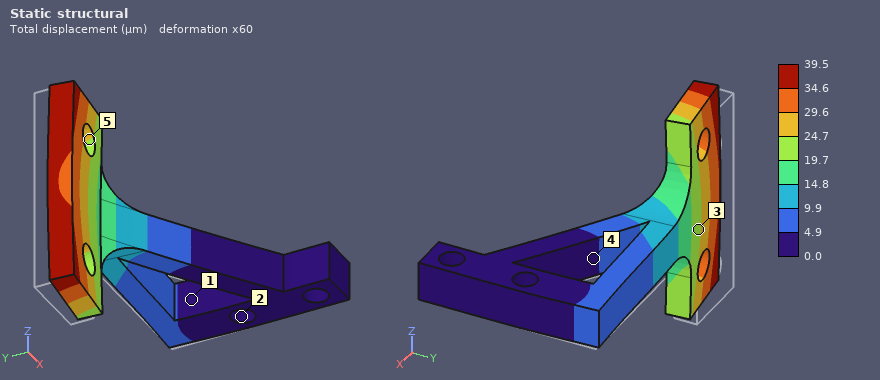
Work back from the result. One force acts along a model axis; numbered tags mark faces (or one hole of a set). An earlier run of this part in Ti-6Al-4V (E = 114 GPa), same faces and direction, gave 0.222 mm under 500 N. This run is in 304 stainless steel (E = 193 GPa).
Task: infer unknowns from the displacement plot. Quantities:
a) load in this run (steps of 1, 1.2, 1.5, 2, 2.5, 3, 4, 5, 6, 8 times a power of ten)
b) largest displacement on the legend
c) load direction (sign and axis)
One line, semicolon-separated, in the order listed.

150 N; 39.5 µm; -Y
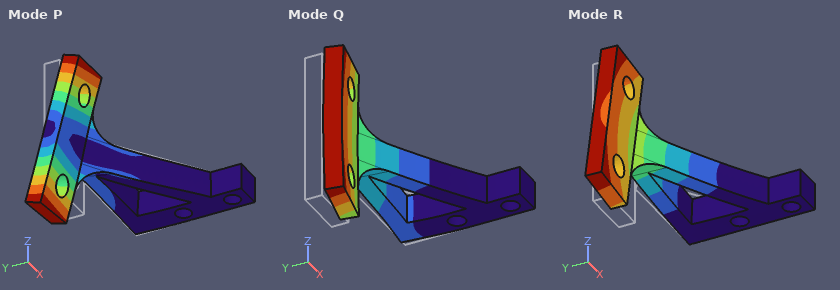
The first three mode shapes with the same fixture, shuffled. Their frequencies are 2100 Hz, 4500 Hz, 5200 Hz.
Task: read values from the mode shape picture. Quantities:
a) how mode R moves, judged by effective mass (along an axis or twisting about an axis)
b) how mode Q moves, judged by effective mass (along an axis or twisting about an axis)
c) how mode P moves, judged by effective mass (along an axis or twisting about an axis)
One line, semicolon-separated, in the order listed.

along Z; along Y; twisting about X
